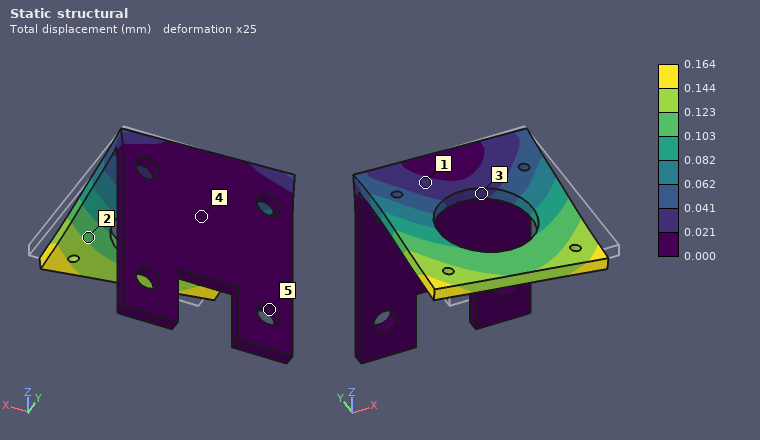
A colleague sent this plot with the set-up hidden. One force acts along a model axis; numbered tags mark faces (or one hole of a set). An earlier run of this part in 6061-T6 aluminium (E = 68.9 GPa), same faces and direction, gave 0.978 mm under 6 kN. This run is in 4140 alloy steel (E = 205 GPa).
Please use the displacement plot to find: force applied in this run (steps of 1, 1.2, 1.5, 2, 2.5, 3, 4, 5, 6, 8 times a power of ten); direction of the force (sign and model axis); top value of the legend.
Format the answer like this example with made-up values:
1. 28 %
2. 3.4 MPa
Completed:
1. 3 kN
2. -X
3. 0.164 mm
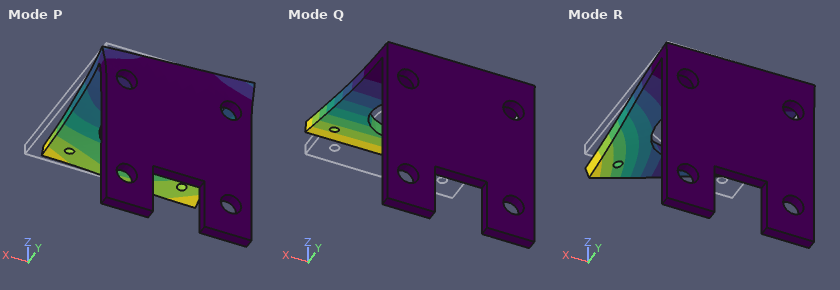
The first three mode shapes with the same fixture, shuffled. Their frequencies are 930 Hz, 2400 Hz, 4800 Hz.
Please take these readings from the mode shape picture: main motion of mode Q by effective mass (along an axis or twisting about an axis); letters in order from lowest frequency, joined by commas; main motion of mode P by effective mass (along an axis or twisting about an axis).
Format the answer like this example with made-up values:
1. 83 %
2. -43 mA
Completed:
1. along Z
2. Q, R, P
3. along X
